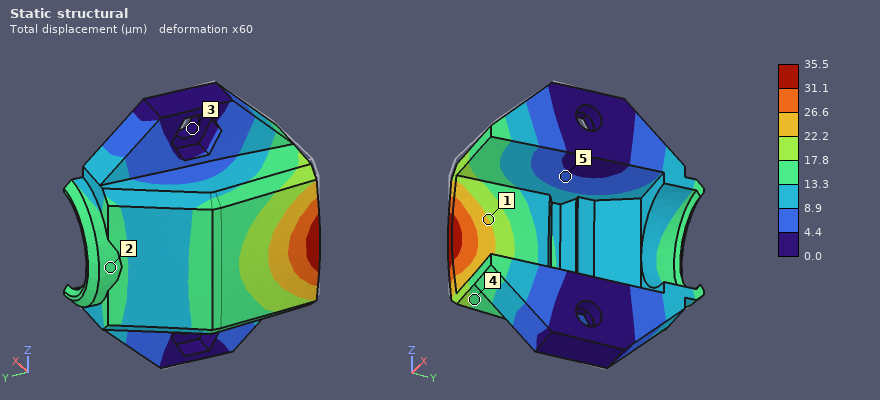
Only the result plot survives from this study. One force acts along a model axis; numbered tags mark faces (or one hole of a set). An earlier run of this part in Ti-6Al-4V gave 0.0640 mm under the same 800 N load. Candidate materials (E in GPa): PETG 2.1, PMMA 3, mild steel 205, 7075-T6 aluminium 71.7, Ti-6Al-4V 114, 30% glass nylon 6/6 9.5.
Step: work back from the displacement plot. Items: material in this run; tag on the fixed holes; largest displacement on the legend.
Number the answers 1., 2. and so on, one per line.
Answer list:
1. mild steel
2. 3
3. 35.5 µm
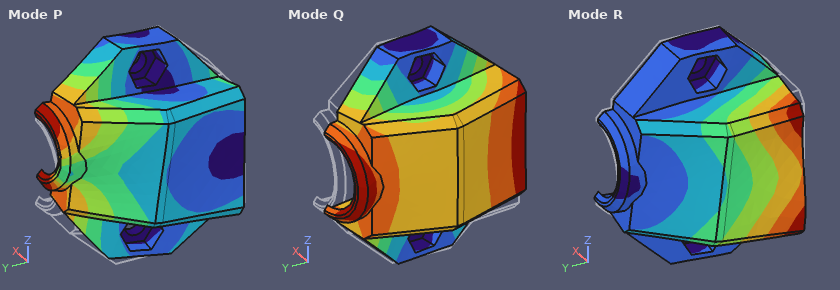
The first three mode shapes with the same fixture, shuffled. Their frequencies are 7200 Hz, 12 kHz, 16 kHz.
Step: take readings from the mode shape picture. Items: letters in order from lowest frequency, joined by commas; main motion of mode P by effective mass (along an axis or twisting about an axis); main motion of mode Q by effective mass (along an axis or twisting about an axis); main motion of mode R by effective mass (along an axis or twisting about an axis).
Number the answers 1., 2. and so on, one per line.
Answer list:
1. Q, R, P
2. along Z
3. along Y
4. along Z
